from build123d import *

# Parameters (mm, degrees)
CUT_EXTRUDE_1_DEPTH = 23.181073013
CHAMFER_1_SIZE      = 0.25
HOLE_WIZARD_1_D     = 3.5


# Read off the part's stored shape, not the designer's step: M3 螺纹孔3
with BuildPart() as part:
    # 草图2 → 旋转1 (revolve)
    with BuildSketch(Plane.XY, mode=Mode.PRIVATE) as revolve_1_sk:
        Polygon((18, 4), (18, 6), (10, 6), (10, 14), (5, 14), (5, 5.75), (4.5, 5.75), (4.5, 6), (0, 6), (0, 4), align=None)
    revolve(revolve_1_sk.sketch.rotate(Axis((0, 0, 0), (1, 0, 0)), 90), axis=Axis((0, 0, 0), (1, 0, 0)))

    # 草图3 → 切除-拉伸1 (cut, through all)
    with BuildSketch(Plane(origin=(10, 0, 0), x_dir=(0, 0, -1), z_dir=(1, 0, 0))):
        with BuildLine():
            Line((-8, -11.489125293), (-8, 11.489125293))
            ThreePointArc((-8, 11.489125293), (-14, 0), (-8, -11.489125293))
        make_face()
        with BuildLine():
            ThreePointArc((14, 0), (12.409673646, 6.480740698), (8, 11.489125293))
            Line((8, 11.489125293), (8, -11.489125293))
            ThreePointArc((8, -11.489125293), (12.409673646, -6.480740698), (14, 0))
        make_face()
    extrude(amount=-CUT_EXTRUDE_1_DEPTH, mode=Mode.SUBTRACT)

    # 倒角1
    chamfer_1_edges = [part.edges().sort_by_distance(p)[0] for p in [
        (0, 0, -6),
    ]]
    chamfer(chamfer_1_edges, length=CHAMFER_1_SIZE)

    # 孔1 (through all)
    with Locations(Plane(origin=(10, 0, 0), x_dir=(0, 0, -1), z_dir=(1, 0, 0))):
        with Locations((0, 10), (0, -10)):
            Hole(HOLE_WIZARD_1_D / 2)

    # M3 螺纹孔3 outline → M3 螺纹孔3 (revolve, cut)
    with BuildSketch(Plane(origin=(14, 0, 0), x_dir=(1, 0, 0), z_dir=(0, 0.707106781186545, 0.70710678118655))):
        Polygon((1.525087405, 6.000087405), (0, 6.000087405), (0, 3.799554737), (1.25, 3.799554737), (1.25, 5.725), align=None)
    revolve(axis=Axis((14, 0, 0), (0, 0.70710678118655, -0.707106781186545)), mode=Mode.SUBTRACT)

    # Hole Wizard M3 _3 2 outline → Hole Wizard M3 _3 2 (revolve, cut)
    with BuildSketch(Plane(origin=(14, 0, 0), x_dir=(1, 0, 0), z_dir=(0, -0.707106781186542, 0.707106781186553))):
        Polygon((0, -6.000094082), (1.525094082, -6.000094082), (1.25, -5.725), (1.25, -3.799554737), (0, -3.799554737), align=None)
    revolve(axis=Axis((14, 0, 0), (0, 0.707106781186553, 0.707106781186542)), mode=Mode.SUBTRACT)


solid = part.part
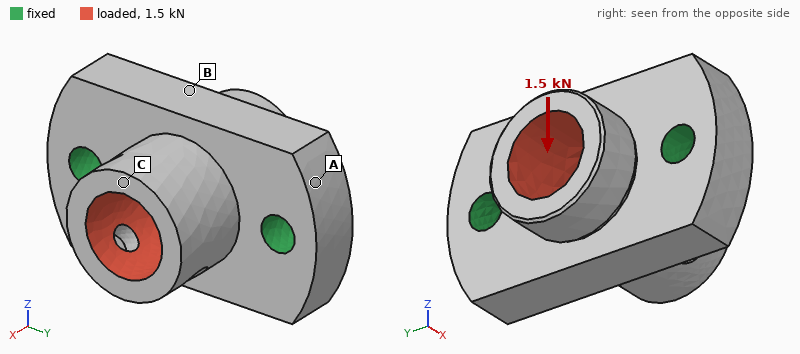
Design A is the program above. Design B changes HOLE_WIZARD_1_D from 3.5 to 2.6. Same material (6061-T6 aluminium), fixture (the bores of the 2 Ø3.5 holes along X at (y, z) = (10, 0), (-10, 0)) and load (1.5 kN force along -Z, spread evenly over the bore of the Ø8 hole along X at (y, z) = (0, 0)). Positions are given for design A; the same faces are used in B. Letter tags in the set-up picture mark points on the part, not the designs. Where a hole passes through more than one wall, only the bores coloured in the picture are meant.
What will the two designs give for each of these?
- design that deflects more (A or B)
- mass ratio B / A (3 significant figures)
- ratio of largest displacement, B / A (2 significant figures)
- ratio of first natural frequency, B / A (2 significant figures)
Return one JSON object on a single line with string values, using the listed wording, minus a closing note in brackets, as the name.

{"design that deflects more": "B", "mass ratio B / A": "1.02", "ratio of largest displacement, B / A": "1.1", "ratio of first natural frequency, B / A": "0.90"}
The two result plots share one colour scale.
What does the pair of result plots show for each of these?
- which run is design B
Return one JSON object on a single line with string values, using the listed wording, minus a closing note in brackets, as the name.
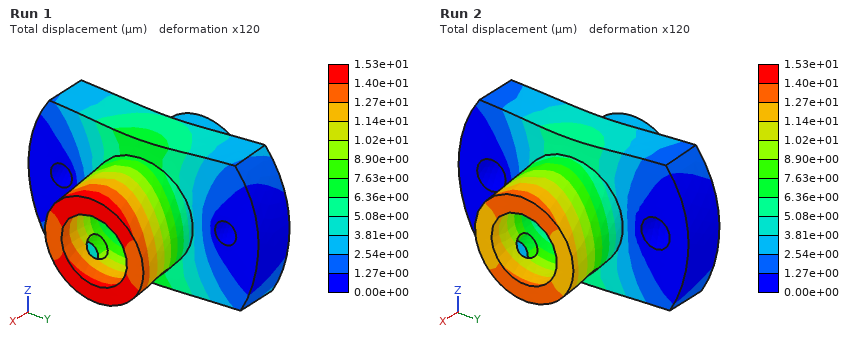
{"which run is design B": "Run 1"}
